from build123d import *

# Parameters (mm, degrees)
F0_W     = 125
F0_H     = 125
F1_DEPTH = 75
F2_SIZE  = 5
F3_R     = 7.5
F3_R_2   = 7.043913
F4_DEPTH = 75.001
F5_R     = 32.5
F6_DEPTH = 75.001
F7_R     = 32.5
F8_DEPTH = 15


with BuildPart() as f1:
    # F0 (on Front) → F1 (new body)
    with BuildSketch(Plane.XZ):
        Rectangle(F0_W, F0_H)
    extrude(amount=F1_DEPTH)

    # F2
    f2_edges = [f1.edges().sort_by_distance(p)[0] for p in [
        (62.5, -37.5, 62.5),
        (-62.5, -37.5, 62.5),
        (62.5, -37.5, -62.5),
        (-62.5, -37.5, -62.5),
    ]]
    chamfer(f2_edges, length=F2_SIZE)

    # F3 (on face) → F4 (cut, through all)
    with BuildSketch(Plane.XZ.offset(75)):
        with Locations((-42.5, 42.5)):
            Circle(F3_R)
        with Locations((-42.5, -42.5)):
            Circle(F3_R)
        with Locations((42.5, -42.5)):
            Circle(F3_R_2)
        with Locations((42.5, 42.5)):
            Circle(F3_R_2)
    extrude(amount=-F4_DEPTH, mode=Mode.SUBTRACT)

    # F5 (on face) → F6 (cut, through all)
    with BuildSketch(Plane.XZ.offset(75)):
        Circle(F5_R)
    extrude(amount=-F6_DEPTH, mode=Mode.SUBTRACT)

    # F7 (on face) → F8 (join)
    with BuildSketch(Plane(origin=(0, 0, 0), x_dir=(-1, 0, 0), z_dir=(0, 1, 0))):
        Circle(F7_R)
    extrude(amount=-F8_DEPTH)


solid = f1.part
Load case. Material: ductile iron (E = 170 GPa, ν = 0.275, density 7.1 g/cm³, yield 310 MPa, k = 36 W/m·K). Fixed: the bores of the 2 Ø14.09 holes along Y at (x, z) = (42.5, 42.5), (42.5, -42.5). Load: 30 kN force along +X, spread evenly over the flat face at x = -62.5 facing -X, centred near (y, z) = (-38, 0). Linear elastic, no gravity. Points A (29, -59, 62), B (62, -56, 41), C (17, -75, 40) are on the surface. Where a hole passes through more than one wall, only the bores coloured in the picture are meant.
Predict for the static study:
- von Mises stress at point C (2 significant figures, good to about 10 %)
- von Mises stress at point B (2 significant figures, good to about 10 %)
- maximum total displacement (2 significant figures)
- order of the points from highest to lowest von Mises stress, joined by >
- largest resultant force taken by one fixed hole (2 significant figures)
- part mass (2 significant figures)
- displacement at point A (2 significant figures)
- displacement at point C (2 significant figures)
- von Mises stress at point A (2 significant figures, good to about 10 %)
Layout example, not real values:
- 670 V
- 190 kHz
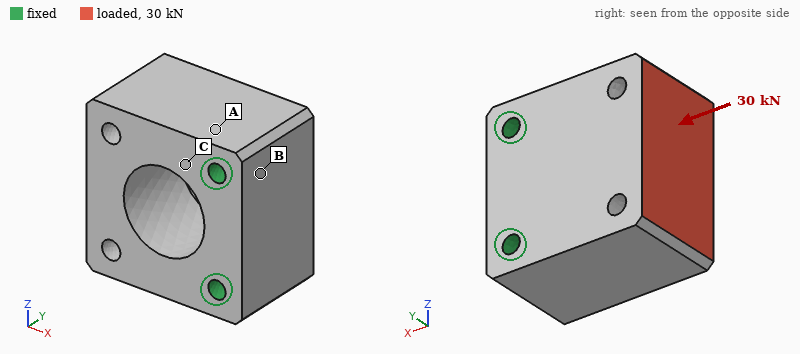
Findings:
- 9.7 MPa
- 1.9 MPa
- 6.8 µm
- C > A > B
- 15 kN
- 6.5 kg
- 1.2 µm
- 1.3 µm
- 5.1 MPa
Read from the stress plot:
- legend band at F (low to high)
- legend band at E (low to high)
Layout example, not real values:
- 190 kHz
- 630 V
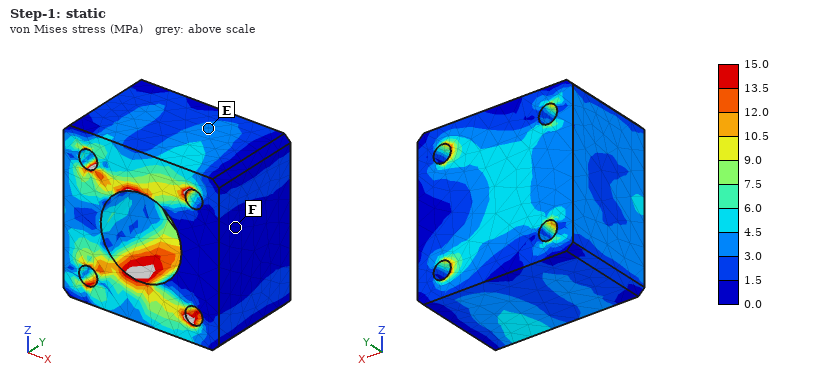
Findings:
- 0.0 to 1.5 MPa
- 3.0 to 4.5 MPa
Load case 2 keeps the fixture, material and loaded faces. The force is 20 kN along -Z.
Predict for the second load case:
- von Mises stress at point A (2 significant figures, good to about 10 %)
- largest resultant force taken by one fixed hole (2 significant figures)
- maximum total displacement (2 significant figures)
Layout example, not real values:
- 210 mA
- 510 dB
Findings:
- 13 MPa
- 23 kN
- 18 µm
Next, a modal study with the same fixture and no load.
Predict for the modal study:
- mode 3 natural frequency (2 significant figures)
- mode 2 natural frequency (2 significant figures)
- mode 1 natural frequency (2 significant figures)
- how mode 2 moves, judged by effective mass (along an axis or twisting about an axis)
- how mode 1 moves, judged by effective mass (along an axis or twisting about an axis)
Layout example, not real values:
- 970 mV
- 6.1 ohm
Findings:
- 5900 Hz
- 3800 Hz
- 3400 Hz
- along Z
- along Y
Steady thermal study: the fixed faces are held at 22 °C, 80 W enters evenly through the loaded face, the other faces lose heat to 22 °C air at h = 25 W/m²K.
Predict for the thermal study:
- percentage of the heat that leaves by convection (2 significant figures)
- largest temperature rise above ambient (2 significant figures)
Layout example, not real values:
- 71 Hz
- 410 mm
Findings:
- 29 %
- 32 K
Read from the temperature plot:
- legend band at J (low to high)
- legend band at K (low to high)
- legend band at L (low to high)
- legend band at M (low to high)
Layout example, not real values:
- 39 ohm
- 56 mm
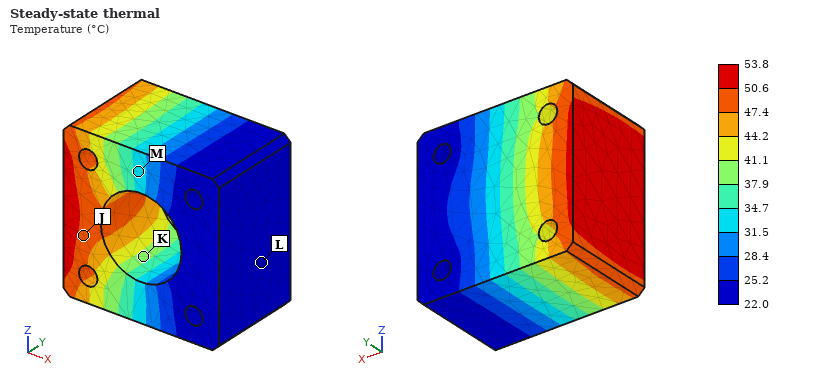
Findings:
- 47.4 to 50.6 °C
- 37.9 to 41.1 °C
- 22.0 to 25.2 °C
- 31.5 to 34.7 °C
